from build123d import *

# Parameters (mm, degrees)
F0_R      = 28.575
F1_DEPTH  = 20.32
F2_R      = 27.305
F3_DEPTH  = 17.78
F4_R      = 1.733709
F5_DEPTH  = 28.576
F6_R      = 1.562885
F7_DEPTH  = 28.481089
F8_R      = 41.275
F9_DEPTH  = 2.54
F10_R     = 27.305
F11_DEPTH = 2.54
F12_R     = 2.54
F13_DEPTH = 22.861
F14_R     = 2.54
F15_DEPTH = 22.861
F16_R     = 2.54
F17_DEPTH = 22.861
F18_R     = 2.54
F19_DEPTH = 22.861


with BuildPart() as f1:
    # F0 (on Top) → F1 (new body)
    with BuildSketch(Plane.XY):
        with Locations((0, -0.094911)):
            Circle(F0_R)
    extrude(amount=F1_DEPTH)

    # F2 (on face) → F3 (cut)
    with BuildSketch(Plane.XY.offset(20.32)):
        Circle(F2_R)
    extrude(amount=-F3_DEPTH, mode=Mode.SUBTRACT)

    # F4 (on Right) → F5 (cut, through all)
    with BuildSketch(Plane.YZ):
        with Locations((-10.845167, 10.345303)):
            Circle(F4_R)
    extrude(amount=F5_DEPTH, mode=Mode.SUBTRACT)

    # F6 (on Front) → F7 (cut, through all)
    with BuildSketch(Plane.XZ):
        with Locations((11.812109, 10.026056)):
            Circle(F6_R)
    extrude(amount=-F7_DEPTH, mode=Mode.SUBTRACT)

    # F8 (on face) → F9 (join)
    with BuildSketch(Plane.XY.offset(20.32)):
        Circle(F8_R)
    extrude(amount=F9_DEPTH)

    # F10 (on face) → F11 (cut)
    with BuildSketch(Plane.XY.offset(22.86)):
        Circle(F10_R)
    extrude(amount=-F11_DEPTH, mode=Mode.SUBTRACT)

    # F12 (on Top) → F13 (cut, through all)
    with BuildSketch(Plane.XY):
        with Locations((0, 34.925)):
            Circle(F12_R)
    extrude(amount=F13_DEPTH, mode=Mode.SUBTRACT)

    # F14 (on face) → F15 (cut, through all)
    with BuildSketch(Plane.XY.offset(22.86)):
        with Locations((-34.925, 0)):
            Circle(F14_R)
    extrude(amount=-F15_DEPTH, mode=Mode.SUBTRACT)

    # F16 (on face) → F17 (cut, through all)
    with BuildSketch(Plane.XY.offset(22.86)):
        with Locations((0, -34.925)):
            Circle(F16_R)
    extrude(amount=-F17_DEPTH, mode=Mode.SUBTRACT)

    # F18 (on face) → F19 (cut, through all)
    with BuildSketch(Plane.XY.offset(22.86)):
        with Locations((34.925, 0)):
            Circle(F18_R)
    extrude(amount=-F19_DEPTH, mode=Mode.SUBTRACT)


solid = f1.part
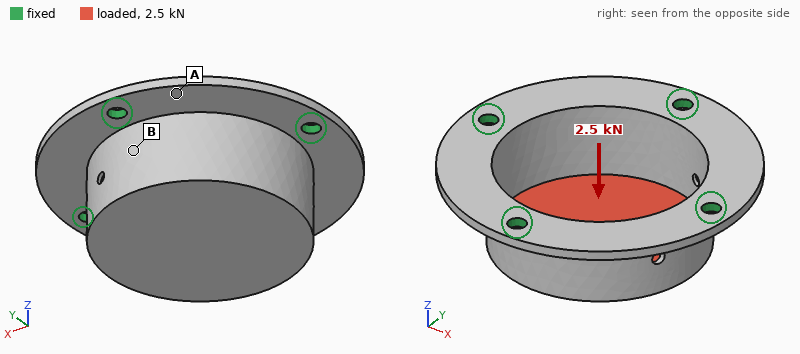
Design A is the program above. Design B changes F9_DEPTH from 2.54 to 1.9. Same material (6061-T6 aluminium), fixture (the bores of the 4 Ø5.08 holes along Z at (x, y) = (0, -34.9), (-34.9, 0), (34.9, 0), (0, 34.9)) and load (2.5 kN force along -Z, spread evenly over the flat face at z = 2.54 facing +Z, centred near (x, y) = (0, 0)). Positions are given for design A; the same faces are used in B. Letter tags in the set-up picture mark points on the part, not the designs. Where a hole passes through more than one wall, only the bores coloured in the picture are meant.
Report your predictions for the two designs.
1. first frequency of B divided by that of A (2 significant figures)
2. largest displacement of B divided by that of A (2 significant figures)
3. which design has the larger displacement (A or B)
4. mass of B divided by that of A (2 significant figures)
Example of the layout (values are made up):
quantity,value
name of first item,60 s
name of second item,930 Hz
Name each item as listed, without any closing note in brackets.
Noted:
quantity,value
first frequency of B divided by that of A,0.92
largest displacement of B divided by that of A,1.1
which design has the larger displacement,B
mass of B divided by that of A,0.90
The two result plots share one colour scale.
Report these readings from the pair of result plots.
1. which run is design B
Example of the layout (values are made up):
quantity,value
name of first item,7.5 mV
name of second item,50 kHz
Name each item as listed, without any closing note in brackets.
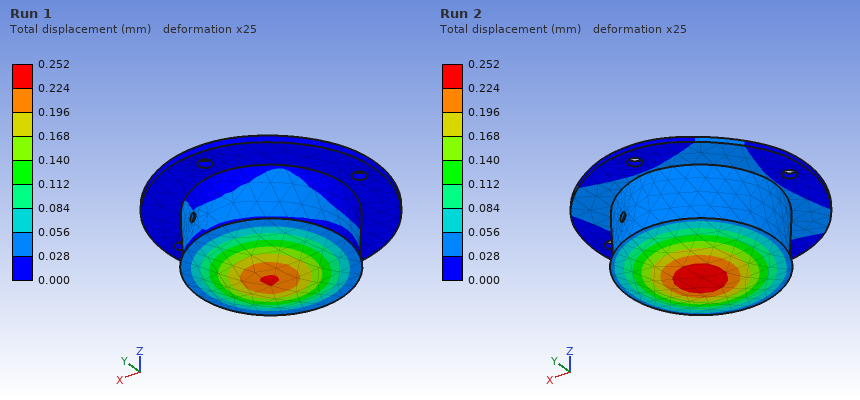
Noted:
quantity,value
which run is design B,Run 2
